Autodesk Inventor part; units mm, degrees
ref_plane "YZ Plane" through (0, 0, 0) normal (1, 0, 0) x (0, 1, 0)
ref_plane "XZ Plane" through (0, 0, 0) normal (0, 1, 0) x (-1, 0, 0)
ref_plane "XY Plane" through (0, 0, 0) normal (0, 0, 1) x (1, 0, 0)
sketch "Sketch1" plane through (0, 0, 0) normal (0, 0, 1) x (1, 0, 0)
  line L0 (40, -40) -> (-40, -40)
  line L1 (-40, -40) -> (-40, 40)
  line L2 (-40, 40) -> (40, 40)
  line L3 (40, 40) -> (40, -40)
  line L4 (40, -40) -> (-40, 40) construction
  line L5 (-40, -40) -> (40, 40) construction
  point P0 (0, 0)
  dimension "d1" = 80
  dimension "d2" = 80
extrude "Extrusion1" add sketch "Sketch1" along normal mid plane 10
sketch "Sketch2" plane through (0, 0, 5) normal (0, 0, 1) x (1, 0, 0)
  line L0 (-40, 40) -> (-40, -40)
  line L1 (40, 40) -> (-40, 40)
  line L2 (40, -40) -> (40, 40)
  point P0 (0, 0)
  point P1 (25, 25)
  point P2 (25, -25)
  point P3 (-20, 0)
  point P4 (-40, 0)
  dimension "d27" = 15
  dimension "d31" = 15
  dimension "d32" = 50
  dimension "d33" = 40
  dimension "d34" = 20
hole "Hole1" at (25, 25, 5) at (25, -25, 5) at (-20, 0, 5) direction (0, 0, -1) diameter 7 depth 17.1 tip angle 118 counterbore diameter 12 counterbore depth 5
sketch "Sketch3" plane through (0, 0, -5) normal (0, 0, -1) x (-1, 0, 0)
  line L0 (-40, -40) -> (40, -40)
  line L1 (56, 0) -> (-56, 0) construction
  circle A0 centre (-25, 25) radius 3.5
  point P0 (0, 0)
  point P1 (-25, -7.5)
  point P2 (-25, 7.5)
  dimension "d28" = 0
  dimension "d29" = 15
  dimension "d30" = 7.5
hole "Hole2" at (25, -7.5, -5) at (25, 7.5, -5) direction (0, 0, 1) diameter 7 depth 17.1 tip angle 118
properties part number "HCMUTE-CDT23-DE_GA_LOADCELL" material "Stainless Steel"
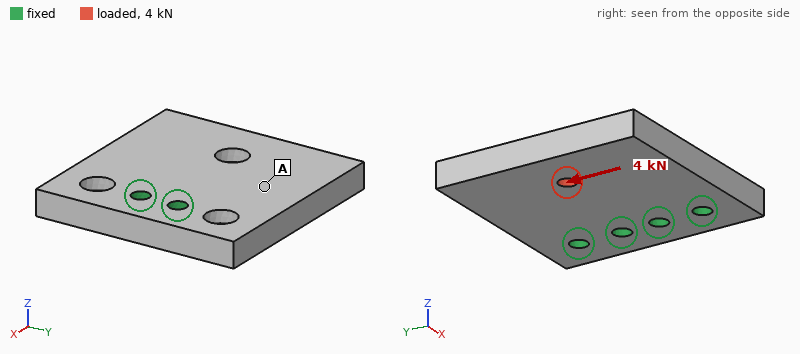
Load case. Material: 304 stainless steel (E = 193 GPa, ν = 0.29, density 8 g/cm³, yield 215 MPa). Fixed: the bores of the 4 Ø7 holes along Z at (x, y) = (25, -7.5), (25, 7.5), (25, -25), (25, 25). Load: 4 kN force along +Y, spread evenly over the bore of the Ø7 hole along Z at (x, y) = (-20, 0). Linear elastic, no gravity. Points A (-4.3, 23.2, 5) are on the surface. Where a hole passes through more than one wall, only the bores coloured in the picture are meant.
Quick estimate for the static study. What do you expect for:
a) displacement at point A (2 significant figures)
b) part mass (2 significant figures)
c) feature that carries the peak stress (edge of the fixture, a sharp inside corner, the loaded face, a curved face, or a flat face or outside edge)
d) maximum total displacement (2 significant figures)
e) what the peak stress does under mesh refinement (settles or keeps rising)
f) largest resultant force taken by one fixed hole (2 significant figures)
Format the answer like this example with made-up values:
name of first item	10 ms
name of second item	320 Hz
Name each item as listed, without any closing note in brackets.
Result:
displacement at point A	5.7 µm
part mass	490 g
feature that carries the peak stress	edge of the fixture
maximum total displacement	15 µm
what the peak stress does under mesh refinement	keeps rising
largest resultant force taken by one fixed hole	3.0 kN
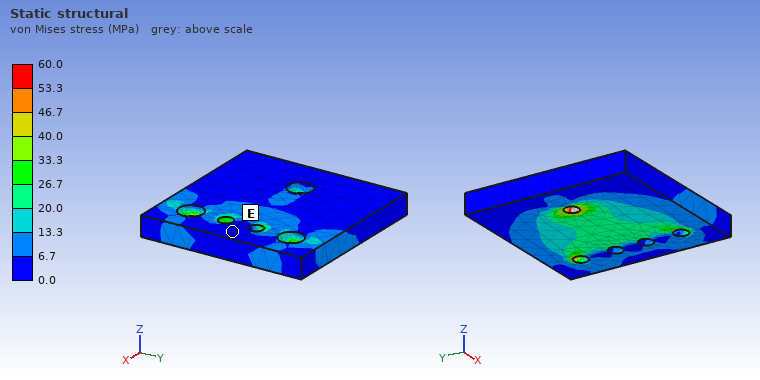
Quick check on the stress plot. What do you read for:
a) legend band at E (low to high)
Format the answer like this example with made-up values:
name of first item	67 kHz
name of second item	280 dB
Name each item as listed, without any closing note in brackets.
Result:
legend band at E	0.0 to 6.7 MPa
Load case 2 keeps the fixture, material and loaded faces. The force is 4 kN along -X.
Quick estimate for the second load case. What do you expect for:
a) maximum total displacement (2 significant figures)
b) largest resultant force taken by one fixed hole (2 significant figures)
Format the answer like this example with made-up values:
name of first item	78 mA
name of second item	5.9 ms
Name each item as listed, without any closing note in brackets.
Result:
maximum total displacement	15 µm
largest resultant force taken by one fixed hole	1.0 kN
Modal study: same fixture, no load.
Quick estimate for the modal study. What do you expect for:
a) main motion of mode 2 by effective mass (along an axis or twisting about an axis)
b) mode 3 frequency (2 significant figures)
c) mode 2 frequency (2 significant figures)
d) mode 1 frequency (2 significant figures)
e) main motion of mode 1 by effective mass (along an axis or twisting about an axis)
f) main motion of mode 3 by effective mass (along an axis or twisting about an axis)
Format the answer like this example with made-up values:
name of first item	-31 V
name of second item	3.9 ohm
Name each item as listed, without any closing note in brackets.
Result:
main motion of mode 2 by effective mass	twisting about X
mode 3 frequency	7000 Hz
mode 2 frequency	3300 Hz
mode 1 frequency	1800 Hz
main motion of mode 1 by effective mass	along Z
main motion of mode 3 by effective mass	along Y
